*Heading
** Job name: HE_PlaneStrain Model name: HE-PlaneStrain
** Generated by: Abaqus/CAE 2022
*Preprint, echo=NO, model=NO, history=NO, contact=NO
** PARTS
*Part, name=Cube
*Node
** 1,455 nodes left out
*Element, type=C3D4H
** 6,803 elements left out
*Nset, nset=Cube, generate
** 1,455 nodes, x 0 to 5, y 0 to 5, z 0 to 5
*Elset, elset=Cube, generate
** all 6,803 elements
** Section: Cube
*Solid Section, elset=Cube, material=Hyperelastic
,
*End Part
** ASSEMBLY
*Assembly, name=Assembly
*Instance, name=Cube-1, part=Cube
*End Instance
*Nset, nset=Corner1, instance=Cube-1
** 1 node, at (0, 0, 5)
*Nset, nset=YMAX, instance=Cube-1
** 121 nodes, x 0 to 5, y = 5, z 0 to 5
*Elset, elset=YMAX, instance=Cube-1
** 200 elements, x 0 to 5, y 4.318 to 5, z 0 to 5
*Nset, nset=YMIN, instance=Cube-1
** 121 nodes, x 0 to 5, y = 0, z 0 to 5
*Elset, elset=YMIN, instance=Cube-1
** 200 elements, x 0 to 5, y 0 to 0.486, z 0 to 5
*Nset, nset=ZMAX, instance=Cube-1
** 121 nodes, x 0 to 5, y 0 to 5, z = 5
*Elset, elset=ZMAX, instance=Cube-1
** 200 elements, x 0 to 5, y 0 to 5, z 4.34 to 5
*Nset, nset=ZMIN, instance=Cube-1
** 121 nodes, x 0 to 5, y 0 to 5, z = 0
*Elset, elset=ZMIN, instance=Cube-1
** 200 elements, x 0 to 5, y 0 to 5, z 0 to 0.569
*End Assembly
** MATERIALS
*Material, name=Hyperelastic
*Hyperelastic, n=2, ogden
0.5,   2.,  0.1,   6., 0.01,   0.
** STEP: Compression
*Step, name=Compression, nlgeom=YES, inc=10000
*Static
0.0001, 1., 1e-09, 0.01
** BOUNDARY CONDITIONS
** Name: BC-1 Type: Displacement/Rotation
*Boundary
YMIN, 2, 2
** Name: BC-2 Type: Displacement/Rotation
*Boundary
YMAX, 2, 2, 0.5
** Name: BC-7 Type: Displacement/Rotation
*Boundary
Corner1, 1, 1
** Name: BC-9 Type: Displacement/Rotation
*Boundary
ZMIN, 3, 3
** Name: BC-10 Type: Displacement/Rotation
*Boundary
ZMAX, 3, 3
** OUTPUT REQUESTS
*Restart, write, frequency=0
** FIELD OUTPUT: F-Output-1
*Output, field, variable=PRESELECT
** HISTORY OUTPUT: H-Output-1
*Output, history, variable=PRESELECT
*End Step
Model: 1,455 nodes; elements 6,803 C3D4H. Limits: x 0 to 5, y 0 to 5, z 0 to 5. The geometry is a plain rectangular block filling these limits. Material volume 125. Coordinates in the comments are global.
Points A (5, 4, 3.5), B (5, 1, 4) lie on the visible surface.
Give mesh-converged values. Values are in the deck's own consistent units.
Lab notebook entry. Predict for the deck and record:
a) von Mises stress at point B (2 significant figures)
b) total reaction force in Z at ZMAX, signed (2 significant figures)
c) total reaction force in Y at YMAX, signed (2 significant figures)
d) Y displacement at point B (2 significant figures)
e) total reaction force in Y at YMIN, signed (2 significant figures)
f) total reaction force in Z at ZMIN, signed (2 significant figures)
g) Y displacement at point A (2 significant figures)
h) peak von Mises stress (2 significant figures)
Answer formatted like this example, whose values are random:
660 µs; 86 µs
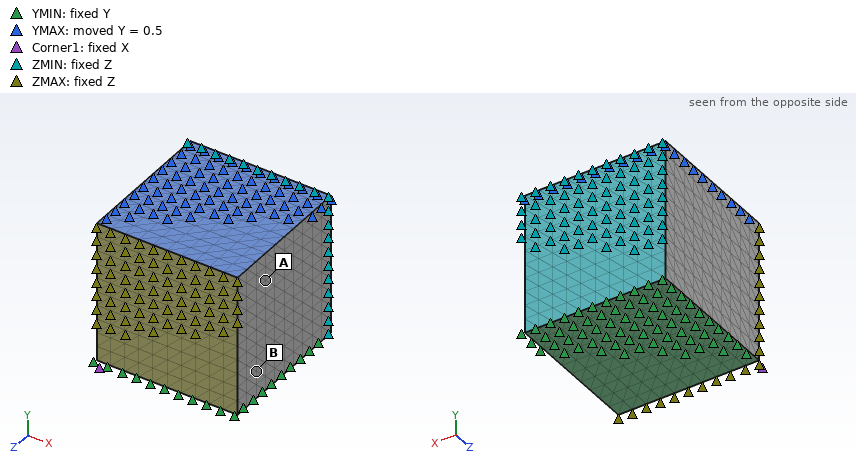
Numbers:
0.16; 2.1; 4.3; 0.10; -4.3; -2.1; 0.40; 0.16
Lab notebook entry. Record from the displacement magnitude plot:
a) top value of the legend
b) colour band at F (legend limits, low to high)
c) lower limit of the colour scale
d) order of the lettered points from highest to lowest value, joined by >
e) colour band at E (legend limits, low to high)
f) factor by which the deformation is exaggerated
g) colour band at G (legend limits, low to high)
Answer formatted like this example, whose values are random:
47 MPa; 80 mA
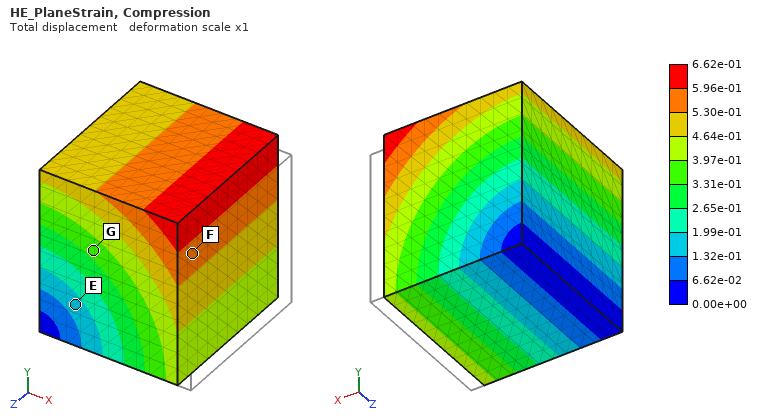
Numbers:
6.62e-01; 5.30e-01 to 5.96e-01; 0.00e+00; F > G > E; 1.32e-01 to 1.99e-01; 1; 3.31e-01 to 3.97e-01
